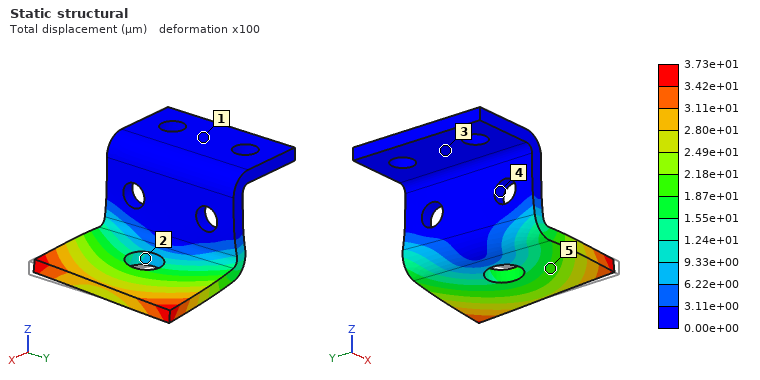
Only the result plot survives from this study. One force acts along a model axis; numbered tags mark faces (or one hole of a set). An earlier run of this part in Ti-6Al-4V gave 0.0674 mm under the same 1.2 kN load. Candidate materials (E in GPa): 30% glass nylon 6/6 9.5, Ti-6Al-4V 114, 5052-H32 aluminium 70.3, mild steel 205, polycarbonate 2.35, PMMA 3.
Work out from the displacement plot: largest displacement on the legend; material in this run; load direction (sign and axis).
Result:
3.73e+01 µm
mild steel
+Y
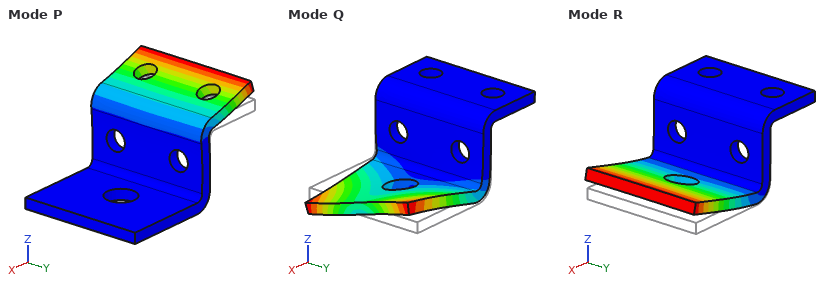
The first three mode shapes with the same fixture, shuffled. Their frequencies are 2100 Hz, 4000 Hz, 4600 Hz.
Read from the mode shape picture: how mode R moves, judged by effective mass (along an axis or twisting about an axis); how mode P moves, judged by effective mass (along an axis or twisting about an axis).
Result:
along Z
along Z
